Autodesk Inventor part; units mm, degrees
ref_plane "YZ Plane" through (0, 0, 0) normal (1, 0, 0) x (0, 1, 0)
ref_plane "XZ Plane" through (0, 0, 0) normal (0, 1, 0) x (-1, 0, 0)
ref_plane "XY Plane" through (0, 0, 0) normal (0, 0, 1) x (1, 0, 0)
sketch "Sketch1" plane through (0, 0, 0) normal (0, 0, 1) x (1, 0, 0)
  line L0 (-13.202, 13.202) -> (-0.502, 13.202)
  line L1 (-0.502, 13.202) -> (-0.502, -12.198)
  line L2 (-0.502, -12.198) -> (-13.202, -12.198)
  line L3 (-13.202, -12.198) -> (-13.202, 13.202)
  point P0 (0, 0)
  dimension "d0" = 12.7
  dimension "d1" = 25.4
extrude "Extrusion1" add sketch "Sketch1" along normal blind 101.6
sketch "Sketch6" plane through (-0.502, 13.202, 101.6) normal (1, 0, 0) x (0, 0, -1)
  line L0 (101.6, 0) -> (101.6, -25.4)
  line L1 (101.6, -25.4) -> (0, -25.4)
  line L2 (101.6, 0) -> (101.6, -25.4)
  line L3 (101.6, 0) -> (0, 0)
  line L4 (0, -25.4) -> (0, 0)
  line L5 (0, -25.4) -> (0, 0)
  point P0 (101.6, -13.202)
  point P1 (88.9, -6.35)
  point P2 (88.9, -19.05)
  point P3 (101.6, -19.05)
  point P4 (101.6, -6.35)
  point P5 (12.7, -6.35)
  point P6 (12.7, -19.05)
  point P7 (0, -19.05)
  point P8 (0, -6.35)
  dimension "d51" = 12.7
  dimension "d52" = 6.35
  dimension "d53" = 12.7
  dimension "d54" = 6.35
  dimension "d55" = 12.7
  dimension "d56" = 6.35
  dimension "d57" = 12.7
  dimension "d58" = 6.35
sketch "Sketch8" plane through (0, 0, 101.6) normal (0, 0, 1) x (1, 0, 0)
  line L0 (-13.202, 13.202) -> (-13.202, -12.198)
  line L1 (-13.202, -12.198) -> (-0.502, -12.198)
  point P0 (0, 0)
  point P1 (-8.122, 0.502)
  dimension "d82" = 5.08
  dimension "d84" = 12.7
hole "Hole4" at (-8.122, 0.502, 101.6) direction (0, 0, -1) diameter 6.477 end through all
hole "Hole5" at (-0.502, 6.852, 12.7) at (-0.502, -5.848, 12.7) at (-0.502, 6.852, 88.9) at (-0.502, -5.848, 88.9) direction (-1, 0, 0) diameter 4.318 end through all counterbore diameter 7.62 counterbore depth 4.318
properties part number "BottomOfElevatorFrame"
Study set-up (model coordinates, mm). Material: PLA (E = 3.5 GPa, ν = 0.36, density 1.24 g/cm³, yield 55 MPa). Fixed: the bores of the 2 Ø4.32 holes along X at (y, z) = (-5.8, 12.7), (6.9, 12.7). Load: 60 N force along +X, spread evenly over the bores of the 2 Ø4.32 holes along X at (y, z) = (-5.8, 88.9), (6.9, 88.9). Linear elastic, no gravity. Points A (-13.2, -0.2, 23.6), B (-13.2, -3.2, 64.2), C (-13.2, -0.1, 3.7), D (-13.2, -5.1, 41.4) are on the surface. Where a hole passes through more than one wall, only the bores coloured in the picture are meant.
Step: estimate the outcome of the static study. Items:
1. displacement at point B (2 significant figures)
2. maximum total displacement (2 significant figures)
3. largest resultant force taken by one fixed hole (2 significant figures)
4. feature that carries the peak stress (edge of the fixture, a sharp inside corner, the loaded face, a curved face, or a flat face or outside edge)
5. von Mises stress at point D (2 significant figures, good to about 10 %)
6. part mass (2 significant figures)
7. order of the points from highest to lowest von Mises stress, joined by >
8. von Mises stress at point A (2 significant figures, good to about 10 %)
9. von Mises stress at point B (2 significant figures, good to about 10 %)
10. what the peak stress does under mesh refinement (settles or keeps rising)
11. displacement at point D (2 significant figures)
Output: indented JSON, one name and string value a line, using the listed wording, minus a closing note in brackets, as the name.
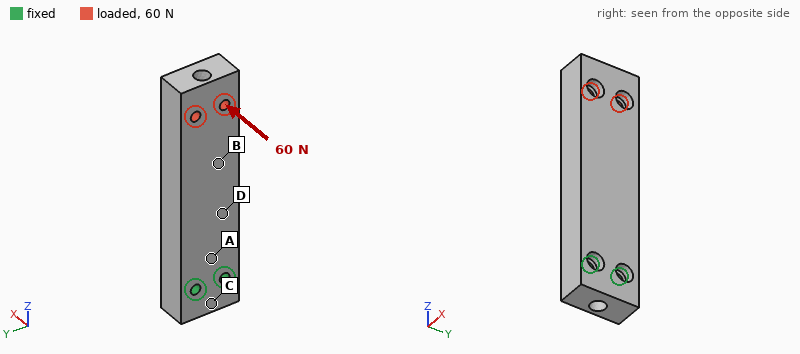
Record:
{
  "displacement at point B": "0.44 mm",
  "maximum total displacement": "0.96 mm",
  "largest resultant force taken by one fixed hole": "33 N",
  "feature that carries the peak stress": "edge of the fixture",
  "von Mises stress at point D": "4.4 MPa",
  "part mass": "35 g",
  "order of the points from highest to lowest von Mises stress, joined by >": "A > D > B > C",
  "von Mises stress at point A": "6.1 MPa",
  "von Mises stress at point B": "2.3 MPa",
  "what the peak stress does under mesh refinement": "keeps rising",
  "displacement at point D": "0.19 mm"
}
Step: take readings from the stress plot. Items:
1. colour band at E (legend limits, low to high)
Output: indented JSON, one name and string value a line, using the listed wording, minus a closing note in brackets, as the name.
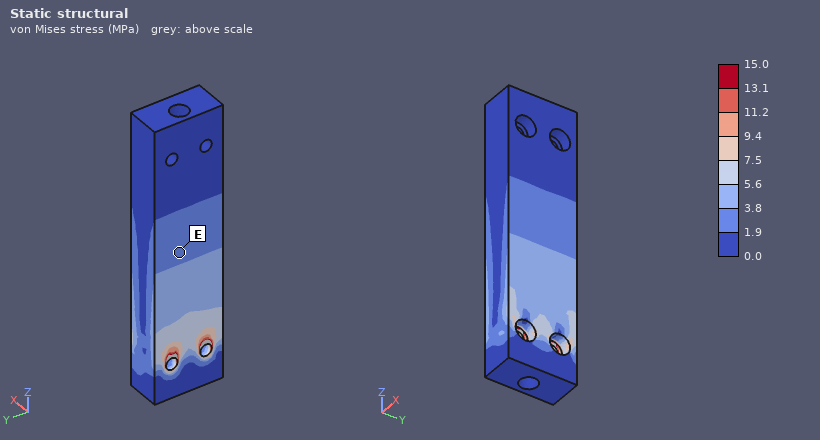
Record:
{
  "colour band at E": "1.9 to 3.8 MPa"
}
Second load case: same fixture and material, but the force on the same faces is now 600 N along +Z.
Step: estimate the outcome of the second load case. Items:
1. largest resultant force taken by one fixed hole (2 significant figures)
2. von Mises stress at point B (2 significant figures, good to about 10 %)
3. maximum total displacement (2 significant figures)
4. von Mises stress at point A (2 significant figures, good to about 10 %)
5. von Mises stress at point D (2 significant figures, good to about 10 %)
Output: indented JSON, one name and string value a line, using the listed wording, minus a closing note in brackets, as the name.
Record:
{
  "largest resultant force taken by one fixed hole": "300 N",
  "von Mises stress at point B": "4.2 MPa",
  "maximum total displacement": "0.34 mm",
  "von Mises stress at point A": "4.2 MPa",
  "von Mises stress at point D": "4.2 MPa"
}
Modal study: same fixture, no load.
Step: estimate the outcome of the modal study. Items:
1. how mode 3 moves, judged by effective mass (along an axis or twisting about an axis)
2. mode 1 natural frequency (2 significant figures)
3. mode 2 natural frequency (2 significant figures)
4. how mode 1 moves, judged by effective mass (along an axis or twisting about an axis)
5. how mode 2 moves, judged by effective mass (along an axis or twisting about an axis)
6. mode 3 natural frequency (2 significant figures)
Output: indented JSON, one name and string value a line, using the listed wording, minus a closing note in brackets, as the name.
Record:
{
  "how mode 3 moves, judged by effective mass": "twisting about Z",
  "mode 1 natural frequency": "400 Hz",
  "mode 2 natural frequency": "790 Hz",
  "how mode 1 moves, judged by effective mass": "along X",
  "how mode 2 moves, judged by effective mass": "along Y",
  "mode 3 natural frequency": "2100 Hz"
}
